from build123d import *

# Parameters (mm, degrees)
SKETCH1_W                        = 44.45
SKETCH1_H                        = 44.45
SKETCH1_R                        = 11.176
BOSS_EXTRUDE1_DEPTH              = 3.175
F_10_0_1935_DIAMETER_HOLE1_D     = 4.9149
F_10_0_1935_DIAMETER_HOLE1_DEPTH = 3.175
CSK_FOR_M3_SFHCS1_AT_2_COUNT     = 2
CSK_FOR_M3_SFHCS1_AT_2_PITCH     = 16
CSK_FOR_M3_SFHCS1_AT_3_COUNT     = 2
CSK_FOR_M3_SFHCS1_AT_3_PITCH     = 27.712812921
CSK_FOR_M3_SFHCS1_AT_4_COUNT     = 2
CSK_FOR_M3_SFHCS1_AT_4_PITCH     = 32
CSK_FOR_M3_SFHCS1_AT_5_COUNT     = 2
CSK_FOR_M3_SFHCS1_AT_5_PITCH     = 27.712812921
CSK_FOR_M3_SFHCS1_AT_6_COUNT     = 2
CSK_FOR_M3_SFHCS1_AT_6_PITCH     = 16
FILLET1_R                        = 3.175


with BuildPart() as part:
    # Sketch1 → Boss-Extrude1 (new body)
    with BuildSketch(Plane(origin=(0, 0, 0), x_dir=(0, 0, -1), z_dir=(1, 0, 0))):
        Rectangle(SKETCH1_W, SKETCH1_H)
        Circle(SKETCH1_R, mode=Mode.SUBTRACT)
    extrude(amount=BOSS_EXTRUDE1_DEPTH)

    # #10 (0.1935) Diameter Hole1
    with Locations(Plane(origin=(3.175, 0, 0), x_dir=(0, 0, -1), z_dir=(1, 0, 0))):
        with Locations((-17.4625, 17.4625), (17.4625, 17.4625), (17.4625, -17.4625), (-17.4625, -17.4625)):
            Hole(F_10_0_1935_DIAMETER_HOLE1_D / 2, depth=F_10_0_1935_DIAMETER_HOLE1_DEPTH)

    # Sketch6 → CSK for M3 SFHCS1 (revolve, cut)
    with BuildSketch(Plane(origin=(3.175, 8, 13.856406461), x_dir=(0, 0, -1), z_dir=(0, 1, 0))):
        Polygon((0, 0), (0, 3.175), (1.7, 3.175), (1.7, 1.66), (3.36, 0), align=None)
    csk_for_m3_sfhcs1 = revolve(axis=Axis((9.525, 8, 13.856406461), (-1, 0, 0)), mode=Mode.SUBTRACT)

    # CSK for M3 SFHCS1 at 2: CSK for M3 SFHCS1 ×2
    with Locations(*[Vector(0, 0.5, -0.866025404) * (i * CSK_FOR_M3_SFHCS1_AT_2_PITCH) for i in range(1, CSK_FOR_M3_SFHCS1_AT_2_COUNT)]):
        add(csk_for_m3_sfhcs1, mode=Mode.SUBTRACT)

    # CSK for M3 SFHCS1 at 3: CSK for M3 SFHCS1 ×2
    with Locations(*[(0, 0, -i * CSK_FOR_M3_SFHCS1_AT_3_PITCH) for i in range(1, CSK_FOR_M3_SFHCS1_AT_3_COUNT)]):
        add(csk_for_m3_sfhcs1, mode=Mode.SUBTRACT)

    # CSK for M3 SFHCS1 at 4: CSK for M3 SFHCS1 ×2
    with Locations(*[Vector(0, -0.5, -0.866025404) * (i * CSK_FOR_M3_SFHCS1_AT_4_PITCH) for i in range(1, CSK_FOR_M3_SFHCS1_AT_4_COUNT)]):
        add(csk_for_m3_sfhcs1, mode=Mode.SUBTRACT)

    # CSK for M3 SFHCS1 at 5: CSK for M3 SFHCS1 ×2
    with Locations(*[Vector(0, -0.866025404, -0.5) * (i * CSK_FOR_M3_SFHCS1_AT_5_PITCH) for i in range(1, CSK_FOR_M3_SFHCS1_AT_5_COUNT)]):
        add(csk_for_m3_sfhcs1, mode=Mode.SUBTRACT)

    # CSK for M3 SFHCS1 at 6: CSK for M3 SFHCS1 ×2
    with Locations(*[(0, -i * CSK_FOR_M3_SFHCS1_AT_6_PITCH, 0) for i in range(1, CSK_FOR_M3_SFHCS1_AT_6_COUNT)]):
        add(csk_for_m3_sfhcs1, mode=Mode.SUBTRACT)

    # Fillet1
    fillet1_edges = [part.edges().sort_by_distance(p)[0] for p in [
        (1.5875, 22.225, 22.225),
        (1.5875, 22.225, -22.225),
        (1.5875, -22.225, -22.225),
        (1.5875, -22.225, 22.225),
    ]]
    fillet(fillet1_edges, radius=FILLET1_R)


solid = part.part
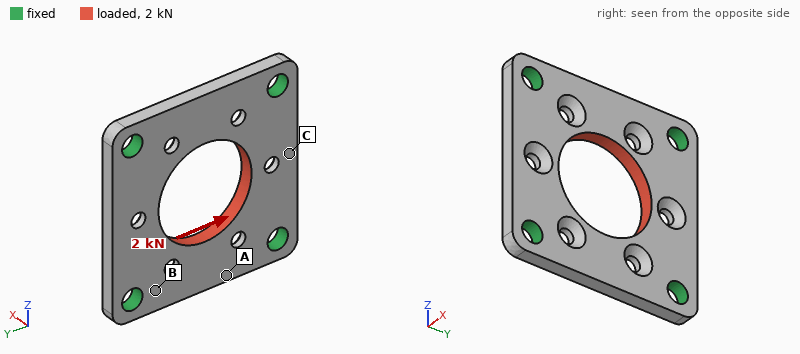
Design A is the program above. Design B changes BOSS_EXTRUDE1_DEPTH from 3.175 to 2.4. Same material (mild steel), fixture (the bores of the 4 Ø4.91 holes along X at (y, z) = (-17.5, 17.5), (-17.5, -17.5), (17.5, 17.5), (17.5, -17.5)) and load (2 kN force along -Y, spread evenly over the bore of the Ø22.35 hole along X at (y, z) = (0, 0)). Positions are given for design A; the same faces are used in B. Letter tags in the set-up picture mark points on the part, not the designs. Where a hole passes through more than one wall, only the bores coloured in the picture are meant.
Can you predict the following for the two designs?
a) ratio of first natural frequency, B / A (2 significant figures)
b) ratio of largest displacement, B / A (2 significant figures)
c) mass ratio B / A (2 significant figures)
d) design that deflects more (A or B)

0.79
1.2
0.77
B
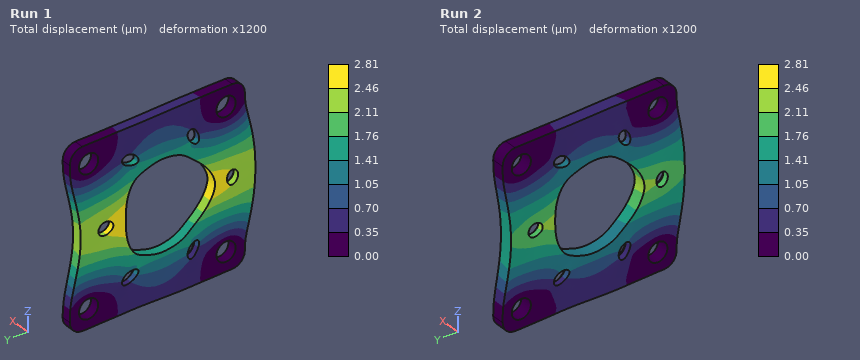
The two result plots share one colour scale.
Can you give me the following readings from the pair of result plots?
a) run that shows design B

Run 1
